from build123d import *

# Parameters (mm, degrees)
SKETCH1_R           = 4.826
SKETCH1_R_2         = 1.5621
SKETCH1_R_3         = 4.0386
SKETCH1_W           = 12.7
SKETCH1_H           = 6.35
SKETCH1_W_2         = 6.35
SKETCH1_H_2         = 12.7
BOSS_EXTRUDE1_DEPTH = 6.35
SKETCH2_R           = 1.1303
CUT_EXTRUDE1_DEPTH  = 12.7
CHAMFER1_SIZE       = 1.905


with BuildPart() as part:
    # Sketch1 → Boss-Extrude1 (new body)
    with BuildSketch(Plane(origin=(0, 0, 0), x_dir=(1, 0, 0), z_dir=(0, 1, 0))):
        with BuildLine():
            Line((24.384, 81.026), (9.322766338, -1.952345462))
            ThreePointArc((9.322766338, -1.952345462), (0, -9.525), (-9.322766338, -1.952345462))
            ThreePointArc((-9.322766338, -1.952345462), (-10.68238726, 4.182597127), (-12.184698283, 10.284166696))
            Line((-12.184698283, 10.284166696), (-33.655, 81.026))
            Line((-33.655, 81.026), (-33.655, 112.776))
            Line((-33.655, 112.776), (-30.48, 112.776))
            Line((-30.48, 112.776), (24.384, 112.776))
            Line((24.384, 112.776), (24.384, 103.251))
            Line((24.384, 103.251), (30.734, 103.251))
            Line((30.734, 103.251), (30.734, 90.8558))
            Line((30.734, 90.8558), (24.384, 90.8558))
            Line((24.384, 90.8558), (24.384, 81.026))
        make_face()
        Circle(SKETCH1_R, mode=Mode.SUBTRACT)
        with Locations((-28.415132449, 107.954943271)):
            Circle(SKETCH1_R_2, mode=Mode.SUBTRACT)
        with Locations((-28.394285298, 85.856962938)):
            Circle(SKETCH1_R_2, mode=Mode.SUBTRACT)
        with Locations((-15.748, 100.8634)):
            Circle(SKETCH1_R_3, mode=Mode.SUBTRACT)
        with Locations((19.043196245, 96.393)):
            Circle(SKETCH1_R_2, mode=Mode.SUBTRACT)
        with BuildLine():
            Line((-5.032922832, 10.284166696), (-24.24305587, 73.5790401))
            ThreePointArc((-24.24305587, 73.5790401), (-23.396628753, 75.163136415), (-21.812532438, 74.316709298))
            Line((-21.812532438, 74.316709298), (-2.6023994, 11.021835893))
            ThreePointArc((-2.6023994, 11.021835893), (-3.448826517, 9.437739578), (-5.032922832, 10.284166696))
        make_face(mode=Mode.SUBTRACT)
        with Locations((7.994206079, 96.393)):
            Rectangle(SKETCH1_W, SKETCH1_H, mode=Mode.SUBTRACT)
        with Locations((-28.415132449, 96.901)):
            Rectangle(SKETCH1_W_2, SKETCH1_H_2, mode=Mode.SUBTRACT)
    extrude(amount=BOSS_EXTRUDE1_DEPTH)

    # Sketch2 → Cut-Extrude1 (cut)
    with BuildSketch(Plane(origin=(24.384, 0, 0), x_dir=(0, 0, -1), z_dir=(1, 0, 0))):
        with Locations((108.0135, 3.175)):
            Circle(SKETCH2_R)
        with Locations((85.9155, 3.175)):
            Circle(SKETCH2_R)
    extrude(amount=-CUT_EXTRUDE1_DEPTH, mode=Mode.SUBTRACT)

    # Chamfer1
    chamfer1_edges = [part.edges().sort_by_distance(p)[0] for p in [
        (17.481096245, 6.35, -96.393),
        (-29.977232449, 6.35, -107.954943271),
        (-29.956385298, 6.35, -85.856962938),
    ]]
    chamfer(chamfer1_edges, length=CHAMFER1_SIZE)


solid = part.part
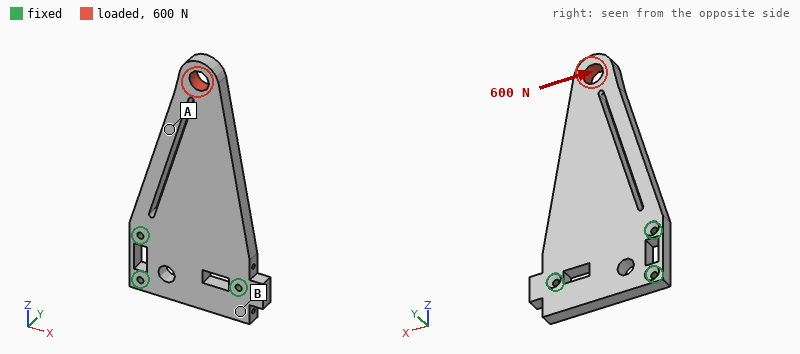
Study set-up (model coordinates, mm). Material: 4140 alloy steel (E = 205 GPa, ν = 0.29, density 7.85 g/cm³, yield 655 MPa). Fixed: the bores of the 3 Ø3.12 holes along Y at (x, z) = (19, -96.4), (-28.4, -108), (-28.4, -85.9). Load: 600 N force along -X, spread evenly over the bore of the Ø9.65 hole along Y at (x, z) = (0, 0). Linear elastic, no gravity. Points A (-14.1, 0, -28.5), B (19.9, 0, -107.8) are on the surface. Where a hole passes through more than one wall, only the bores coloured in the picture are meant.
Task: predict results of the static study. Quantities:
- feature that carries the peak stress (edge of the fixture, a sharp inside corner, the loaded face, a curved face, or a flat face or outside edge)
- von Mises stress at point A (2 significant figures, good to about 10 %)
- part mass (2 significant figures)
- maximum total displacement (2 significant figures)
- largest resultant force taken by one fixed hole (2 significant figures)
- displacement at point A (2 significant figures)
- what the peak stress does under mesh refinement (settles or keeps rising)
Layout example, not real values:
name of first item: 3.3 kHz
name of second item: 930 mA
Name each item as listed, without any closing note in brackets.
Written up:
feature that carries the peak stress: edge of the fixture
von Mises stress at point A: 13 MPa
part mass: 230 g
maximum total displacement: 23 µm
largest resultant force taken by one fixed hole: 1.1 kN
displacement at point A: 11 µm
what the peak stress does under mesh refinement: keeps rising
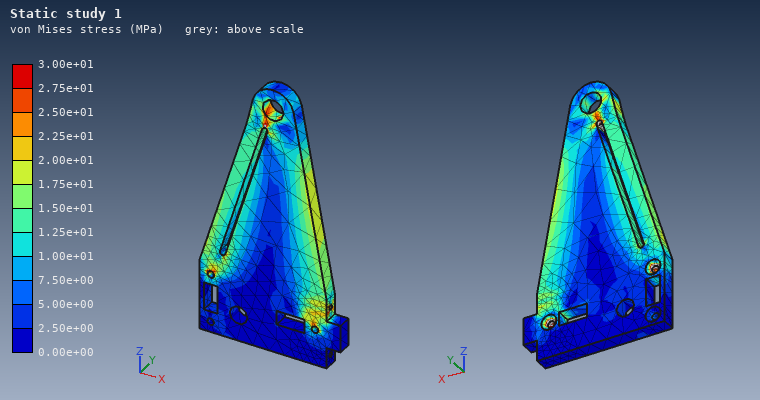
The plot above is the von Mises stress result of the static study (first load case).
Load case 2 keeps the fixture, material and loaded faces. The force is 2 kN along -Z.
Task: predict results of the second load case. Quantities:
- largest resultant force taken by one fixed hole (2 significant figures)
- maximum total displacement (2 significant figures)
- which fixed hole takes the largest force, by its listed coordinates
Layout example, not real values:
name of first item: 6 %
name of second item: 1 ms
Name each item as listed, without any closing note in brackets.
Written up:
largest resultant force taken by one fixed hole: 1.2 kN
maximum total displacement: 9.1 µm
which fixed hole takes the largest force, by its listed coordinates: (19, -96.4)
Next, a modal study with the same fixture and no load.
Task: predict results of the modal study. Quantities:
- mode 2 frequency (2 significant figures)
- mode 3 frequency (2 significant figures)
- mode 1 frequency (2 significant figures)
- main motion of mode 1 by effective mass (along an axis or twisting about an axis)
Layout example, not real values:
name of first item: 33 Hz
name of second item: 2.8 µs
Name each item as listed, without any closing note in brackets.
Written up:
mode 2 frequency: 3100 Hz
mode 3 frequency: 3800 Hz
mode 1 frequency: 710 Hz
main motion of mode 1 by effective mass: along Y
